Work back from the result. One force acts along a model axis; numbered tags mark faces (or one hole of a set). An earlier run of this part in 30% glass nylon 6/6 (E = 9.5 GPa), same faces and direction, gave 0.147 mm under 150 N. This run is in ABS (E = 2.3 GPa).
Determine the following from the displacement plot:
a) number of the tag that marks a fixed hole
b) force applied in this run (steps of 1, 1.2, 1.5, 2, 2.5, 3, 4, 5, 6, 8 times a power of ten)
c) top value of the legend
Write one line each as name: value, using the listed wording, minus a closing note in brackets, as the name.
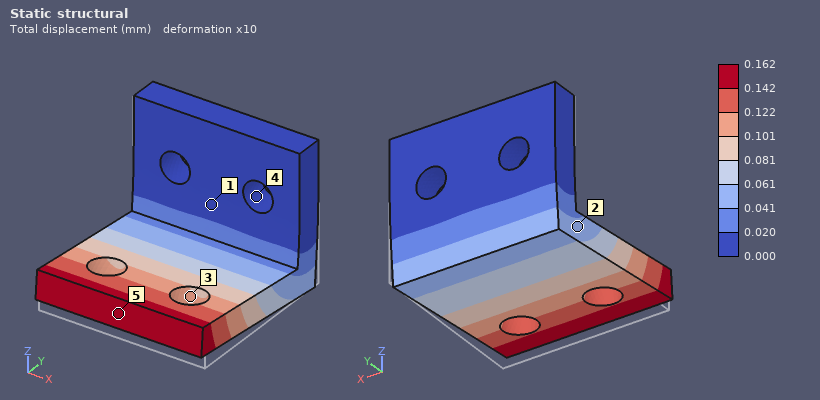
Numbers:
number of the tag that marks a fixed hole: 4
force applied in this run: 40 N
top value of the legend: 0.162 mm
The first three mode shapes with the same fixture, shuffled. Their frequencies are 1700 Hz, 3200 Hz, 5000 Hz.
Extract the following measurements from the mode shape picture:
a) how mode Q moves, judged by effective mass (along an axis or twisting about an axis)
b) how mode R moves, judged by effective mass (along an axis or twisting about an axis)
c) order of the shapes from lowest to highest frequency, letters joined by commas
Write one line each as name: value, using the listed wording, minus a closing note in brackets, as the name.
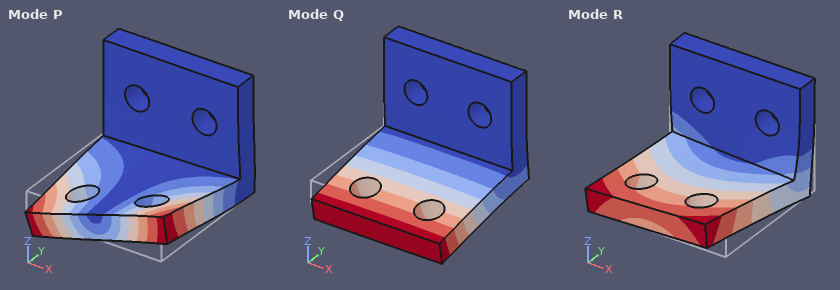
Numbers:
how mode Q moves, judged by effective mass: along Z
how mode R moves, judged by effective mass: along X
order of the shapes from lowest to highest frequency, letters joined by commas: Q, R, P
